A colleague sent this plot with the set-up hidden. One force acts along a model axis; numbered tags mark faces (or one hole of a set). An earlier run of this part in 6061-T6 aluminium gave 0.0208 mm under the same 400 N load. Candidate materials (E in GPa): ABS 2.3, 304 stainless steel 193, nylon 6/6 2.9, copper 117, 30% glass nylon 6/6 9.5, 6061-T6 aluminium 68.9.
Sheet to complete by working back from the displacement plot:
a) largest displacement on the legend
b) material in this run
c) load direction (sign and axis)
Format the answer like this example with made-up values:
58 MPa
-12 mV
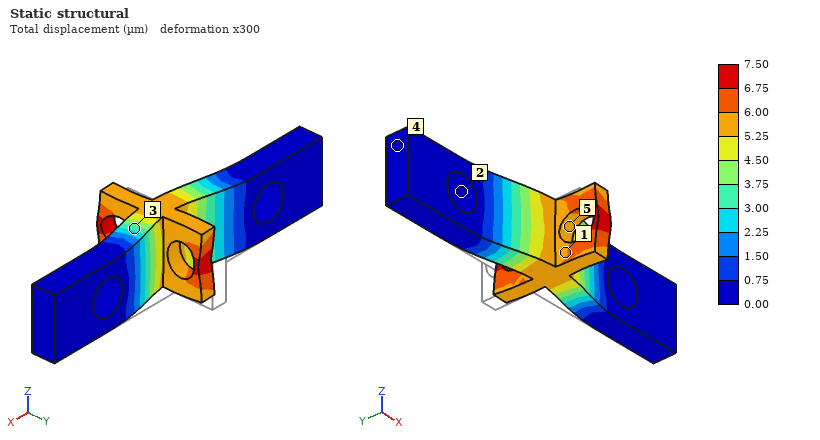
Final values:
7.50 µm
304 stainless steel
-Y
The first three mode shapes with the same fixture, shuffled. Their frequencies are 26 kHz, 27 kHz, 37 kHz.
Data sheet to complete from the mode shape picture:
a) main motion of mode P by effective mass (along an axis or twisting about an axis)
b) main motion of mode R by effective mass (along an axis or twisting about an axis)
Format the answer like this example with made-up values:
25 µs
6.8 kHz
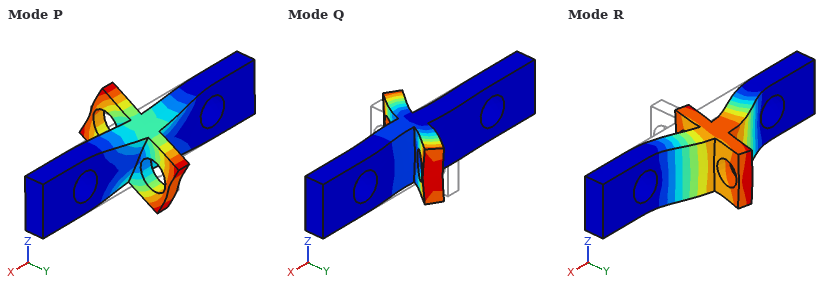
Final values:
twisting about X
along Y
